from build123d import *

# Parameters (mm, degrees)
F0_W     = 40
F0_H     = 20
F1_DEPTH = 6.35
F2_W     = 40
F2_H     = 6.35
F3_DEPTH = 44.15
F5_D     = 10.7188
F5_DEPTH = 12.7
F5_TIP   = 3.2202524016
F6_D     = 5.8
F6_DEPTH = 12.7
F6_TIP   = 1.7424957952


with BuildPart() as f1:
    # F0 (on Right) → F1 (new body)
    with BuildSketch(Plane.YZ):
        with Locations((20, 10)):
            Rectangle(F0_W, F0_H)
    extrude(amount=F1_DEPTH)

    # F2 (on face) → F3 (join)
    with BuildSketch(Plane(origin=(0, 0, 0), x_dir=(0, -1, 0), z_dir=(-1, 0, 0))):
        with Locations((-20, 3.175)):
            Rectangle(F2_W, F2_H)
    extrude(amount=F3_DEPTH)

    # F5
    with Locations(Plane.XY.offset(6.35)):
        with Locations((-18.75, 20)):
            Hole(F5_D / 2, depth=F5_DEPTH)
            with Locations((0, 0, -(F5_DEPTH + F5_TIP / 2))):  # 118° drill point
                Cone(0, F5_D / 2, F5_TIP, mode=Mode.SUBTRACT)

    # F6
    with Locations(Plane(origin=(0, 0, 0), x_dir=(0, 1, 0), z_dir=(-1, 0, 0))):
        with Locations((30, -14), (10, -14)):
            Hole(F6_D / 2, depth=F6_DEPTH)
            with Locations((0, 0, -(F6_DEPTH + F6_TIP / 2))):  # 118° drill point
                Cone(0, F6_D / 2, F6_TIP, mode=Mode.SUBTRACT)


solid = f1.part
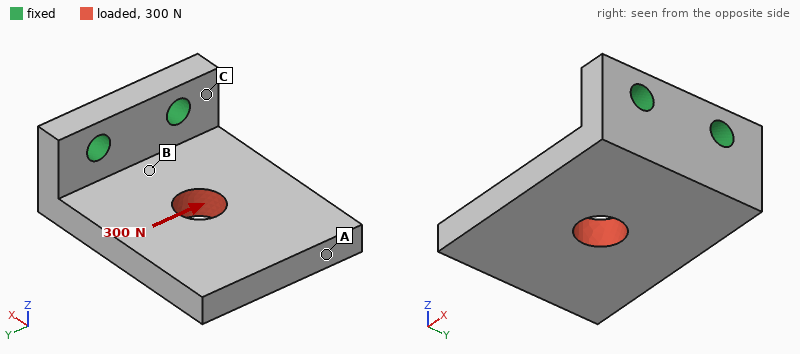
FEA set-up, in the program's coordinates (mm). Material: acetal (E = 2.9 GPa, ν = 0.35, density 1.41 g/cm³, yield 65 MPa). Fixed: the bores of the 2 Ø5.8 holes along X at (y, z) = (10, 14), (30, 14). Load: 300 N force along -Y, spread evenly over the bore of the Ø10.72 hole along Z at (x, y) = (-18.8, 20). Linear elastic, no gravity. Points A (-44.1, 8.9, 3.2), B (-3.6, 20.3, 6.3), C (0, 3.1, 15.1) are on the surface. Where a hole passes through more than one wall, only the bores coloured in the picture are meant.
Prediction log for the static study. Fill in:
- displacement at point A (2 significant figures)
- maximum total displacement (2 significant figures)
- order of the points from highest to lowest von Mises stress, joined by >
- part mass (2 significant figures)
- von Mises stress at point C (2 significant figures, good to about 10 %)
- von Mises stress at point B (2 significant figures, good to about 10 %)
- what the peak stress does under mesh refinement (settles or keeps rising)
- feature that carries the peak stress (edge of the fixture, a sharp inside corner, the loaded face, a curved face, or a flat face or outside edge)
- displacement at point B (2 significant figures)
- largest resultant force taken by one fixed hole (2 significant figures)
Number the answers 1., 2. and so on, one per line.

1. 0.31 mm
2. 0.34 mm
3. B > C > A
4. 22 g
5. 3.9 MPa
6. 6.8 MPa
7. keeps rising
8. edge of the fixture
9. 0.055 mm
10. 320 N
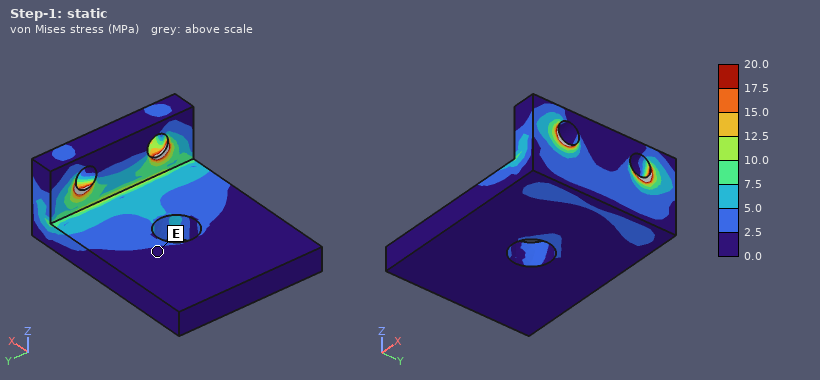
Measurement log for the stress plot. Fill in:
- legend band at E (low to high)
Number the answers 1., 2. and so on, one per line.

1. 0.0 to 2.5 MPa
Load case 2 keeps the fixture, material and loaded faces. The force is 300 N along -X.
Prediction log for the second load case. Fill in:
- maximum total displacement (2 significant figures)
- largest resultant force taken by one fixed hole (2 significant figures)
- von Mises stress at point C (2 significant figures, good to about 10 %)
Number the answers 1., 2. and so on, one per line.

1. 0.32 mm
2. 150 N
3. 2.6 MPa
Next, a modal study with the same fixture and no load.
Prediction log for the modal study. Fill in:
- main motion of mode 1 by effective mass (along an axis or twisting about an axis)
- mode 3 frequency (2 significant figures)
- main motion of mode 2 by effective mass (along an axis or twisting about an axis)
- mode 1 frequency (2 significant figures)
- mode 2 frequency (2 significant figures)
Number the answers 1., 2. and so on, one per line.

1. along Z
2. 1700 Hz
3. along Y
4. 510 Hz
5. 1300 Hz
